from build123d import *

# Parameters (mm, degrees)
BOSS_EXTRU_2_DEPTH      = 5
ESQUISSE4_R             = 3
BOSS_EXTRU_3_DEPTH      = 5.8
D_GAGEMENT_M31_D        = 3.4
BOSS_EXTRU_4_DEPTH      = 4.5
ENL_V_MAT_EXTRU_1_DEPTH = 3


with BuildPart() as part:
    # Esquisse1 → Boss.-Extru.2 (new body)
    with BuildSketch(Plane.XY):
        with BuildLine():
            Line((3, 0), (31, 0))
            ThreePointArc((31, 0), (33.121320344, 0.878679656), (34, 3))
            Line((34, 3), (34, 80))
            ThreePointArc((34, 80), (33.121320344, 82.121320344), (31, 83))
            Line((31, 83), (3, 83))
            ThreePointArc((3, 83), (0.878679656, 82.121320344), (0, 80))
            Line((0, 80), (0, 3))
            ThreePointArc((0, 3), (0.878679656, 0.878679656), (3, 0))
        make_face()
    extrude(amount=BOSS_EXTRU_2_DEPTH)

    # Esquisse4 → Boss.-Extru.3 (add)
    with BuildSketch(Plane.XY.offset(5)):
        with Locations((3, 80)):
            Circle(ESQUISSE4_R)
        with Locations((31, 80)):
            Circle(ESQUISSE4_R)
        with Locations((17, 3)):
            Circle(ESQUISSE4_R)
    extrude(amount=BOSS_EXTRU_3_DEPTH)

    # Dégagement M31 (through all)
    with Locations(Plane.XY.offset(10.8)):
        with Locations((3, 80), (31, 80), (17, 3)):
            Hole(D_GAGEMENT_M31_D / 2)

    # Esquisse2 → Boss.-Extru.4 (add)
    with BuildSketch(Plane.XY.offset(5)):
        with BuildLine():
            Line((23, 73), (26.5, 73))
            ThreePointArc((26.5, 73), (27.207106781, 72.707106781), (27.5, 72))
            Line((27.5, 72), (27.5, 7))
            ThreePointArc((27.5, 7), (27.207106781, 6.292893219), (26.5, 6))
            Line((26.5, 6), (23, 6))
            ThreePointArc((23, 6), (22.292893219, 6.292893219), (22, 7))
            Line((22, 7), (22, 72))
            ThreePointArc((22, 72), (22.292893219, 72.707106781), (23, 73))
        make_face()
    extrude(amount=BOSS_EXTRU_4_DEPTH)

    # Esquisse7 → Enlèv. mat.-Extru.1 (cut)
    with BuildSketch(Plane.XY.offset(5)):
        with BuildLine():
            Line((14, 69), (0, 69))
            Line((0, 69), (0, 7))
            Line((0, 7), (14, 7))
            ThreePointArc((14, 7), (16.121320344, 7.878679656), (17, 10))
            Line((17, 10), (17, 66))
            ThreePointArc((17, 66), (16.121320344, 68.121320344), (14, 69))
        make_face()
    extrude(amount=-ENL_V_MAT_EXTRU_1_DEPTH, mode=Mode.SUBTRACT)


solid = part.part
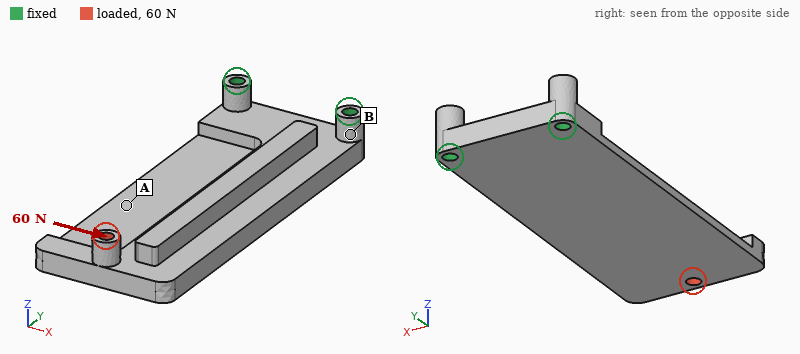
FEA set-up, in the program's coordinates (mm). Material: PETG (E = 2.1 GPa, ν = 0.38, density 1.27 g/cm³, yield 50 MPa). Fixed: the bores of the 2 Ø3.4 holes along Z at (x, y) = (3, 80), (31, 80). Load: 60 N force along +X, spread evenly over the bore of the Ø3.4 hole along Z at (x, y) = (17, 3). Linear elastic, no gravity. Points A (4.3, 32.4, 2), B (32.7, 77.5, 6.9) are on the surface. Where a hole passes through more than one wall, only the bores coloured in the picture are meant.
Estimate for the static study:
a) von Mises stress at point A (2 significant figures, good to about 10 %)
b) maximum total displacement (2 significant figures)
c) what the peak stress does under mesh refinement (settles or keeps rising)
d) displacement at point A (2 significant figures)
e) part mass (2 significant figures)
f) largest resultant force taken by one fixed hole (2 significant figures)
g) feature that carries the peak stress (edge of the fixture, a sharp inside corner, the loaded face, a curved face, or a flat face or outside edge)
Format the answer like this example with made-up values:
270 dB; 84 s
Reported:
3.4 MPa; 1.00 mm; keeps rising; 0.26 mm; 16 g; 170 N; edge of the fixture
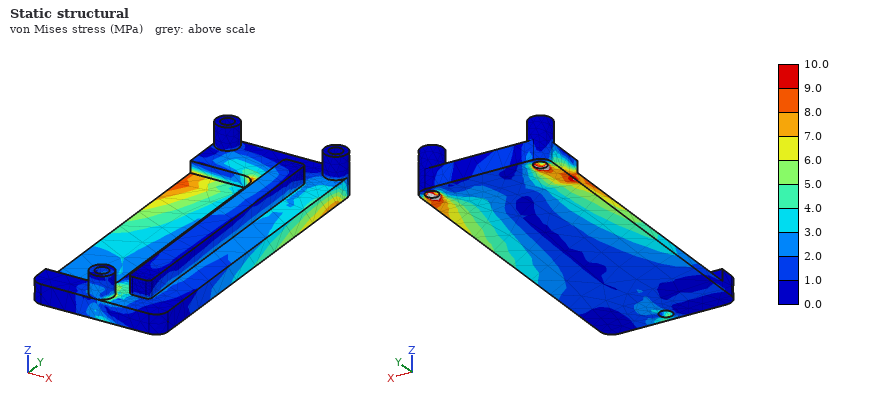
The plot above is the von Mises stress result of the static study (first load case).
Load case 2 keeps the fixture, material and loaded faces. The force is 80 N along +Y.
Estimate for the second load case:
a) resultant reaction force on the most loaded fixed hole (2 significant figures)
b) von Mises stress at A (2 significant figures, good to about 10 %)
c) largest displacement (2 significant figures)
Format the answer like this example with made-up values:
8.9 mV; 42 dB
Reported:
43 N; 1.3 MPa; 0.92 mm
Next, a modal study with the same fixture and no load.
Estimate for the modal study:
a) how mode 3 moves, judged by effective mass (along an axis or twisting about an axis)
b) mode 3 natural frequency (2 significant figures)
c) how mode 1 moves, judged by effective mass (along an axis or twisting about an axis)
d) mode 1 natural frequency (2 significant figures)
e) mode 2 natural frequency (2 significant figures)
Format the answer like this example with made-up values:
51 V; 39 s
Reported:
along X; 850 Hz; along Z; 170 Hz; 700 Hz
